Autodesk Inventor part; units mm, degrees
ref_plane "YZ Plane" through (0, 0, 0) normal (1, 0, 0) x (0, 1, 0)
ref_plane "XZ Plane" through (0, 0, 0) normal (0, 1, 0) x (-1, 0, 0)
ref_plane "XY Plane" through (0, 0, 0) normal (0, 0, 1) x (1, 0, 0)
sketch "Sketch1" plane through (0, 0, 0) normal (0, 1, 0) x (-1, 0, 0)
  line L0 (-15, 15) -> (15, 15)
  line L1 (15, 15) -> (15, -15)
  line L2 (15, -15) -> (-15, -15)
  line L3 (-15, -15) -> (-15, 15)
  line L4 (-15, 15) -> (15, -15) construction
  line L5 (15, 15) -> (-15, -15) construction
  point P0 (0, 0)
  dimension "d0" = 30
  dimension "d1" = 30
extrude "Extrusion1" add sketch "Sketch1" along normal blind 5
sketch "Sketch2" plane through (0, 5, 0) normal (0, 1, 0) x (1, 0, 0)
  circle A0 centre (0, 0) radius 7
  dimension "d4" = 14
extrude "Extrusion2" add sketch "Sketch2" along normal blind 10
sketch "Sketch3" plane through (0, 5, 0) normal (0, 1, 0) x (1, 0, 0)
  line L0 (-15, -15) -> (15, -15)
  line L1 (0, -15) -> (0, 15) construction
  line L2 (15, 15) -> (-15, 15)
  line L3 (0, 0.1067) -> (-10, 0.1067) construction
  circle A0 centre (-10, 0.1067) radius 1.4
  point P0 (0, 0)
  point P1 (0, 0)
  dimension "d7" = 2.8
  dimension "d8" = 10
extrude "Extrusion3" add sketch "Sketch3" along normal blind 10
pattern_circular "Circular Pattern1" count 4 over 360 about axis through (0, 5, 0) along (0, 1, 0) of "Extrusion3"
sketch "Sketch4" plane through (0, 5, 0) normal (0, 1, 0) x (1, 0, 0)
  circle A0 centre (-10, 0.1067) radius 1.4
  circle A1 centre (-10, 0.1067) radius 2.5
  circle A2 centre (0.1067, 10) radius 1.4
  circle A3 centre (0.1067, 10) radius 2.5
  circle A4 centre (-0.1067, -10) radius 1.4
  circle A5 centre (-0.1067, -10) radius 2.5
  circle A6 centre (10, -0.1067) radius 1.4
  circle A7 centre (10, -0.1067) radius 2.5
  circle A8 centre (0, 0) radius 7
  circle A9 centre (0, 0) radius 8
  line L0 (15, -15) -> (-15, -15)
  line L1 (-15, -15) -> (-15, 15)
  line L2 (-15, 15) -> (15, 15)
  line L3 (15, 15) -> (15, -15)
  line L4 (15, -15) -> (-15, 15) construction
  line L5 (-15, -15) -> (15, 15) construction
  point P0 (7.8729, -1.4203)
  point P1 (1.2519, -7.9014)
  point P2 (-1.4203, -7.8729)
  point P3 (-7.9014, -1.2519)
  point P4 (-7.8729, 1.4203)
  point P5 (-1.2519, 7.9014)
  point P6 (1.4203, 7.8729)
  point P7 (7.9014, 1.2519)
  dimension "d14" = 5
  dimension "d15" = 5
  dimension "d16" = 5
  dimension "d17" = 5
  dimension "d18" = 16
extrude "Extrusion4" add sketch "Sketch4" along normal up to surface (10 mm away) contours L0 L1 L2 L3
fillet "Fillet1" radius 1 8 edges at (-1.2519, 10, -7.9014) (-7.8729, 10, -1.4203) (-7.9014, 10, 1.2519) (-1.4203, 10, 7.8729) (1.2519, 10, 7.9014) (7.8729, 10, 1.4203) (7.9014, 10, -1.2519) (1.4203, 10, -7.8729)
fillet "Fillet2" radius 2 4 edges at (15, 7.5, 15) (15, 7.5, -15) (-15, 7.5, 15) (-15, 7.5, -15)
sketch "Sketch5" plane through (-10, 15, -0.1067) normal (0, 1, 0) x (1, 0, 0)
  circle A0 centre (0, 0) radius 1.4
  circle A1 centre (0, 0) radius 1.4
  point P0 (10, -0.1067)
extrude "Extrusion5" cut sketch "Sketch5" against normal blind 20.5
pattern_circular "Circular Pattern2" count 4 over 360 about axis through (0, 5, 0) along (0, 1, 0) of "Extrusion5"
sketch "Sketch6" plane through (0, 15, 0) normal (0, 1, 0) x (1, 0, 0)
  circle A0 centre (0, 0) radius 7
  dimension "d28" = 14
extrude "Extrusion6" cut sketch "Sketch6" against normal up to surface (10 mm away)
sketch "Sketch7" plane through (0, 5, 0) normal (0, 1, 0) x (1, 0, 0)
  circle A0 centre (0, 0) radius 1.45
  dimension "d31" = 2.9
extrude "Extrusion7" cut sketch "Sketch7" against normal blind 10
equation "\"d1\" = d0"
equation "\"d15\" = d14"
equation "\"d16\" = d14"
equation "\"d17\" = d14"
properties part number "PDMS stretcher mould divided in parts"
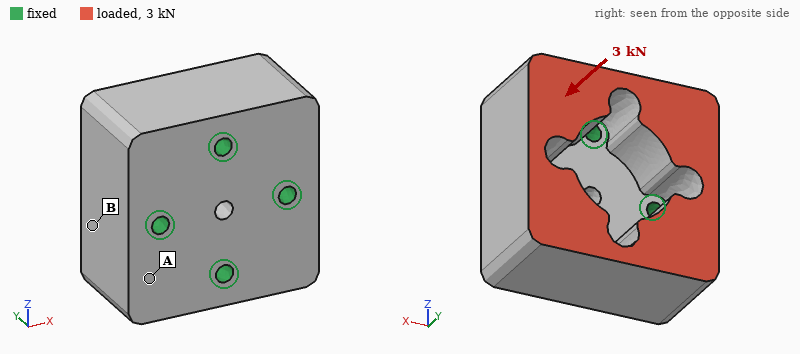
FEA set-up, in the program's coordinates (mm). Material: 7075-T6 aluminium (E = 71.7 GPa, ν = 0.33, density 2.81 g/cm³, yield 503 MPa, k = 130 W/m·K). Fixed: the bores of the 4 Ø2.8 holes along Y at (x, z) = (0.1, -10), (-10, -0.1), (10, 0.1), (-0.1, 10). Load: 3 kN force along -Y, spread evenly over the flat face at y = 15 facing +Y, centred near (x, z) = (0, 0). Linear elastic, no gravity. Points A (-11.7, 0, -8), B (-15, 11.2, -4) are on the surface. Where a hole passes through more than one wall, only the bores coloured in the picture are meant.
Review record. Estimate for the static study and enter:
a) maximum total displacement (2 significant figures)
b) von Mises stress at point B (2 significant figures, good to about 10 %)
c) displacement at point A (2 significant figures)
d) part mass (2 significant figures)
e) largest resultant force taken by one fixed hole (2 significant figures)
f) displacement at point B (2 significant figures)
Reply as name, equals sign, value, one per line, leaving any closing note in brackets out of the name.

maximum total displacement = 4.7 µm
von Mises stress at point B = 11 MPa
displacement at point A = 2.5 µm
part mass = 29 g
largest resultant force taken by one fixed hole = 750 N
displacement at point B = 2.8 µm
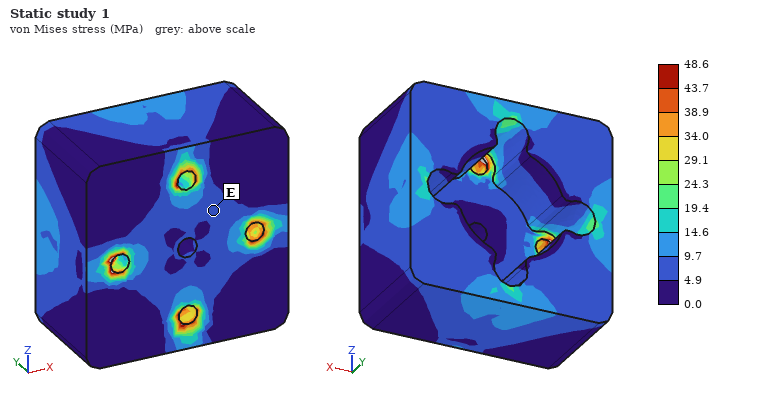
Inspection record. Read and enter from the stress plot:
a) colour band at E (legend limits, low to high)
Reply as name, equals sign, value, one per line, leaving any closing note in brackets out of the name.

colour band at E = 4.9 to 9.7 MPa
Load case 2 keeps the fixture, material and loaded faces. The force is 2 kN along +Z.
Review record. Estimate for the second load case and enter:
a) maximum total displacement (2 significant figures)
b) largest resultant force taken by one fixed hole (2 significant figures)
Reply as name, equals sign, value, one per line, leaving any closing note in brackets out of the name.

maximum total displacement = 13 µm
largest resultant force taken by one fixed hole = 970 N
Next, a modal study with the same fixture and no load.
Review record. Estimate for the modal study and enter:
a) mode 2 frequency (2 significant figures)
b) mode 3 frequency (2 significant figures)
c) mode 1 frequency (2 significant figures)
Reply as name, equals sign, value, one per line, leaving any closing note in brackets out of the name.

mode 2 frequency = 21 kHz
mode 3 frequency = 21 kHz
mode 1 frequency = 21 kHz
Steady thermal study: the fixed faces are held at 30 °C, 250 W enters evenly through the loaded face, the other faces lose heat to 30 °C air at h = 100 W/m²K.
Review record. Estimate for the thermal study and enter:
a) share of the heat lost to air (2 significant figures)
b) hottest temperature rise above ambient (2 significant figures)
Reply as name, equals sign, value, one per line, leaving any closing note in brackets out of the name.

share of the heat lost to air = 4.5 %
hottest temperature rise above ambient = 58 K
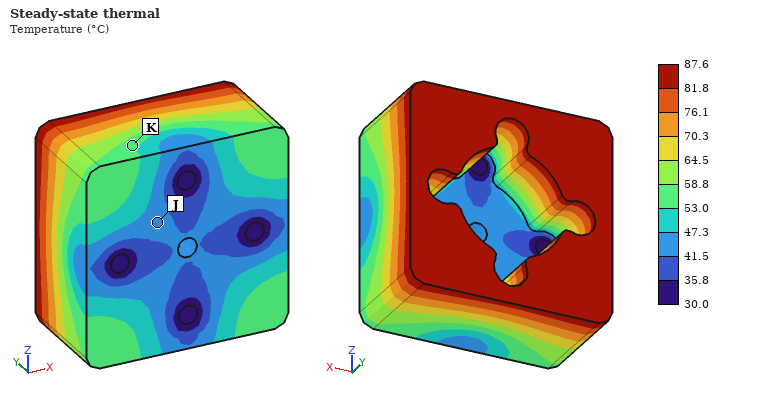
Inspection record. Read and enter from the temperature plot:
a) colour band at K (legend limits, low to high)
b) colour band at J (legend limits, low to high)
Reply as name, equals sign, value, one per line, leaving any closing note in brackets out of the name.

colour band at K = 53.0 to 58.8 °C
colour band at J = 41.5 to 47.3 °C
